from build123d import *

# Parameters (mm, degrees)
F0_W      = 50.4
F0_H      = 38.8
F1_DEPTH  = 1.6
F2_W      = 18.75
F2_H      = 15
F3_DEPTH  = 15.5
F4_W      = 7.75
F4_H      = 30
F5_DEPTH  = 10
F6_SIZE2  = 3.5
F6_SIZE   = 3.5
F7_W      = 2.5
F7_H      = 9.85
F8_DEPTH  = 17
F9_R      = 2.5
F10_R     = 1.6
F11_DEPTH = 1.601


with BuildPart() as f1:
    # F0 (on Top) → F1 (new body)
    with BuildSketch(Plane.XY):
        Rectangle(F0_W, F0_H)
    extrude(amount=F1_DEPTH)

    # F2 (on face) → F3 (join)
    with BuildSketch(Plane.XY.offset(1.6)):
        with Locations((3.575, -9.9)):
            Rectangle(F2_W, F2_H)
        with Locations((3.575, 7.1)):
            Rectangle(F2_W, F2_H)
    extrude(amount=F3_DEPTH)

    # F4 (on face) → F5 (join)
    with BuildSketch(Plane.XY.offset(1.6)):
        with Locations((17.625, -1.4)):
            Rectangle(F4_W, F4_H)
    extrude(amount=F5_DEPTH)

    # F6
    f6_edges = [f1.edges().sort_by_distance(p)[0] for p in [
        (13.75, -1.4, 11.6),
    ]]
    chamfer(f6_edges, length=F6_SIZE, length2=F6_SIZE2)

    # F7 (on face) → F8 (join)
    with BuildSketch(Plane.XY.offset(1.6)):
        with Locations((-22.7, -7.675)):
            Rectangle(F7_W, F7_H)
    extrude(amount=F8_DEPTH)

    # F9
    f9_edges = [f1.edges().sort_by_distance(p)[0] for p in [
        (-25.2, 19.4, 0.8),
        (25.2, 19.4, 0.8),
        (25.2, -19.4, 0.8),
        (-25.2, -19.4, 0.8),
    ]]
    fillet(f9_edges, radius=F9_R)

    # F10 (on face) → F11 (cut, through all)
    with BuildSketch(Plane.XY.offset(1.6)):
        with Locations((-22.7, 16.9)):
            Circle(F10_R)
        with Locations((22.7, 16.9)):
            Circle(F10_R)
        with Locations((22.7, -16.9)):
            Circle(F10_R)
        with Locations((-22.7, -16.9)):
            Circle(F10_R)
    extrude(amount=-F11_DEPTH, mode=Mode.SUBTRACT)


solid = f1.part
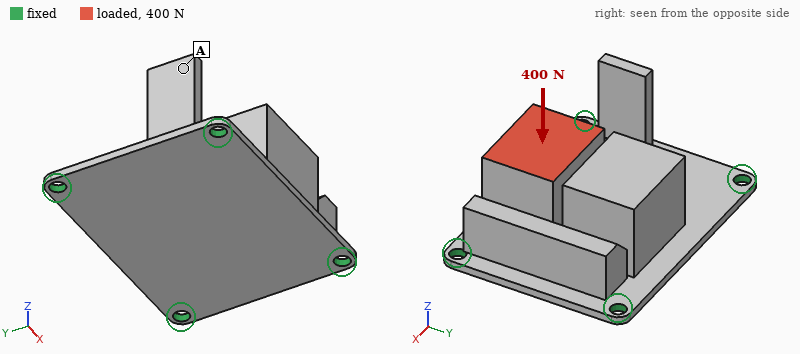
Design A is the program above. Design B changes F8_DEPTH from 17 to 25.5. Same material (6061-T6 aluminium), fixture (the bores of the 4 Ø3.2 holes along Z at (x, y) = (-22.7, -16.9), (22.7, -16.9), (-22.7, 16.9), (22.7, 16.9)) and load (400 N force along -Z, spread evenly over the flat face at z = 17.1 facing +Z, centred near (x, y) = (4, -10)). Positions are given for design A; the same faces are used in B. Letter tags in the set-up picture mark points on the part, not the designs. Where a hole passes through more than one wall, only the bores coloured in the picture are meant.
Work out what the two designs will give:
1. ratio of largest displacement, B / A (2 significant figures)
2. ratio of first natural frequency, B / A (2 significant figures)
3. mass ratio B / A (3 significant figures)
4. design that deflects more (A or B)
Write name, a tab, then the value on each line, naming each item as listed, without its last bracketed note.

ratio of largest displacement, B / A	1.2
ratio of first natural frequency, B / A	0.91
mass ratio B / A	1.01
design that deflects more	B
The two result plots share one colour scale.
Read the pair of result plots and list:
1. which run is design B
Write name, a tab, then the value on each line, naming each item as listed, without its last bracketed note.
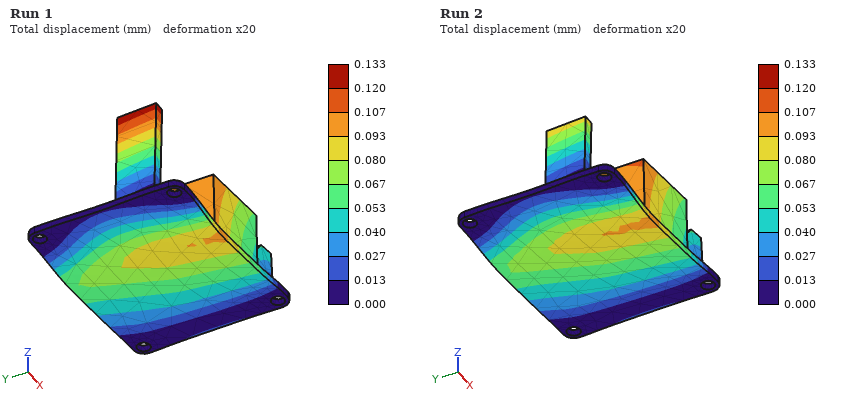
which run is design B	Run 1
